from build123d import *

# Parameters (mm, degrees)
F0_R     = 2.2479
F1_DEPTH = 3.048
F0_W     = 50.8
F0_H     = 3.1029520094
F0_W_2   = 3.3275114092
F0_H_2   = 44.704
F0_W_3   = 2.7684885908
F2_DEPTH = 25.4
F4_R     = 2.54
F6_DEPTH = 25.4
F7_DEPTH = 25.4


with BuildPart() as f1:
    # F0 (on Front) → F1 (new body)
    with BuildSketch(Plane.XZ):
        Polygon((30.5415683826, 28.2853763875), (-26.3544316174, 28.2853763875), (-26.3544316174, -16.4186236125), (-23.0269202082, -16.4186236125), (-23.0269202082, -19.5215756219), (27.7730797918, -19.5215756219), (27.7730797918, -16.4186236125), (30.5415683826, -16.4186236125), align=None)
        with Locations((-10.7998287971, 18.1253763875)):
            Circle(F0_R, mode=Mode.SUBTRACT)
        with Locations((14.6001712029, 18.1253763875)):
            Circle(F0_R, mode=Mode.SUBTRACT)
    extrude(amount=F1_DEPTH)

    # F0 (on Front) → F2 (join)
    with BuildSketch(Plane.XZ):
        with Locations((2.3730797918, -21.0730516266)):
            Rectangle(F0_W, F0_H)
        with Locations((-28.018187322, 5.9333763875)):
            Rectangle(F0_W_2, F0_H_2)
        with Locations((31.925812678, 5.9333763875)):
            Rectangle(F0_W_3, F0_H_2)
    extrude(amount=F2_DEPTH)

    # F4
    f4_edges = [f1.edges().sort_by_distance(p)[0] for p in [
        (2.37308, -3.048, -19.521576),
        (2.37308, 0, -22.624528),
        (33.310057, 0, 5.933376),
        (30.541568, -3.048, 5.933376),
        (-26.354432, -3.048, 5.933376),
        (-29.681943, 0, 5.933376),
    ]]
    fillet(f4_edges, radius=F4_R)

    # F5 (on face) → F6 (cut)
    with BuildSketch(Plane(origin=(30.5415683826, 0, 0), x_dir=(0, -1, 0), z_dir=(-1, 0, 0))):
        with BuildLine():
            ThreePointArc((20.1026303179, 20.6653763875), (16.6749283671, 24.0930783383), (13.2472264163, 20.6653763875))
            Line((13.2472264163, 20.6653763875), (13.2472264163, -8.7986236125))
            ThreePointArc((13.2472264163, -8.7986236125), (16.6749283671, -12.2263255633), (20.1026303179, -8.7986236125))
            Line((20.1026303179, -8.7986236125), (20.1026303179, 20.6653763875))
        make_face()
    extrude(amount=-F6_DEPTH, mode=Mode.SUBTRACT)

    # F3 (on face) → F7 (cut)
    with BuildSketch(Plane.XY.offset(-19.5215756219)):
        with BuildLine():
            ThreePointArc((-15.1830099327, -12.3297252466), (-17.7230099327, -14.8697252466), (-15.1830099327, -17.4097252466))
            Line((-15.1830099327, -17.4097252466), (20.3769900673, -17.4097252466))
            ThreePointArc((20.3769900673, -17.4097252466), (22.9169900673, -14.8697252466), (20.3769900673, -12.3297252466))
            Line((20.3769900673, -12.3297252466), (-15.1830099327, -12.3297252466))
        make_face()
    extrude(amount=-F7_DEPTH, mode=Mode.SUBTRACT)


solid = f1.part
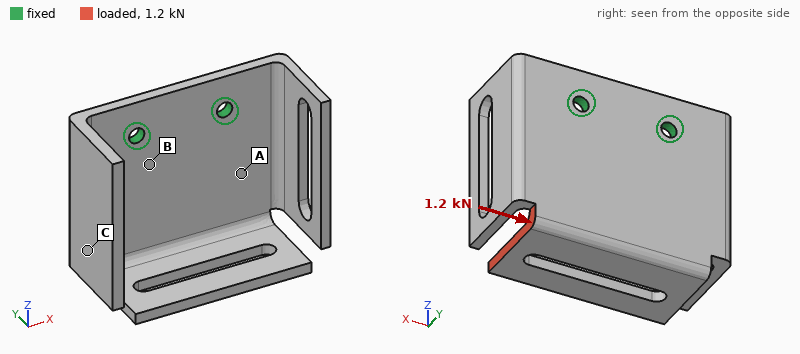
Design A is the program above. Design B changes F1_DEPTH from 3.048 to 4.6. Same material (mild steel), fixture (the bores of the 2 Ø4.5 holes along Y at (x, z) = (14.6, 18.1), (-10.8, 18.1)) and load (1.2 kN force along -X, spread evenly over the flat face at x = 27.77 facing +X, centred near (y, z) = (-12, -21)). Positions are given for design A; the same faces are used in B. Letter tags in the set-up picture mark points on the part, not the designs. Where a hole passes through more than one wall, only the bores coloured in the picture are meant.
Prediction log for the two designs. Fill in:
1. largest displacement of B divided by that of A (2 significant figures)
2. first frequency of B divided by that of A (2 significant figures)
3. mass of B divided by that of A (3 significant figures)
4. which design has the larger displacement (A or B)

0.35
1.6
1.23
A
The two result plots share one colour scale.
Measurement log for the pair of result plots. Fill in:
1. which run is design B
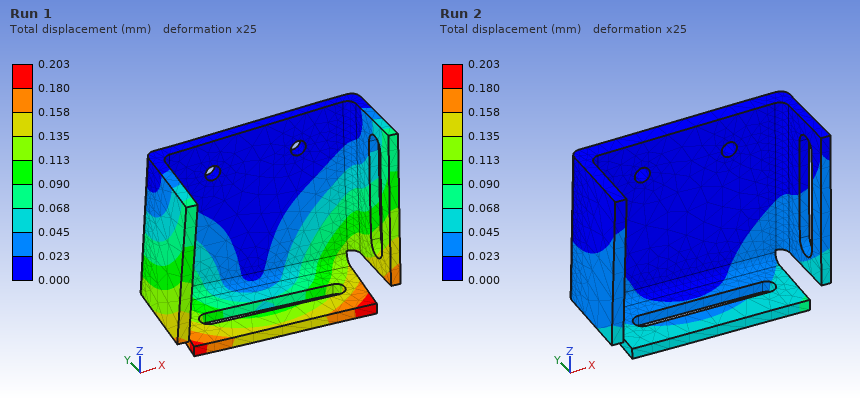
Run 2
